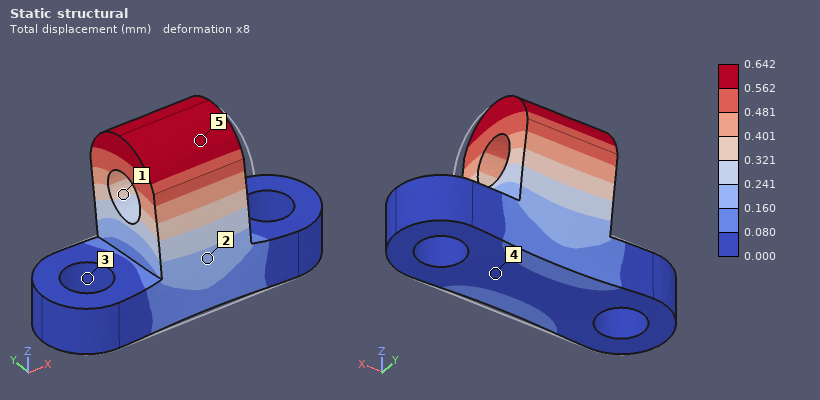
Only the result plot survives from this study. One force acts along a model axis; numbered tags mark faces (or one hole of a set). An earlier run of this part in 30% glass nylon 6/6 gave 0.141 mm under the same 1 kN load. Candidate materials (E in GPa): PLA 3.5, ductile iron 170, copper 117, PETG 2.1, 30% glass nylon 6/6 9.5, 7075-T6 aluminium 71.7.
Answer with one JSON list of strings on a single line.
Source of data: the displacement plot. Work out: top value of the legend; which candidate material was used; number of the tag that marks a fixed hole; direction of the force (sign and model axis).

["0.642 mm", "PETG", "3", "+Y"]
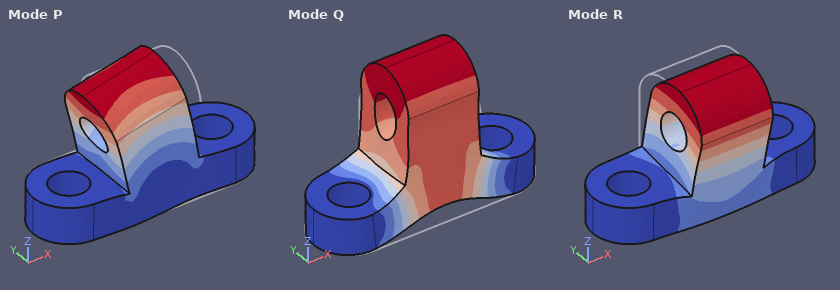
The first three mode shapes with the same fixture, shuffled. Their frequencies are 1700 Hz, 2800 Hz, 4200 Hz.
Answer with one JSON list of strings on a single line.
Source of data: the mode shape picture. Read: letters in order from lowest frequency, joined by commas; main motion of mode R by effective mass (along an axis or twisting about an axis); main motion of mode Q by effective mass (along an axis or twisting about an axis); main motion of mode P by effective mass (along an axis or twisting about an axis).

["R, P, Q", "along Y", "along Z", "along X"]
